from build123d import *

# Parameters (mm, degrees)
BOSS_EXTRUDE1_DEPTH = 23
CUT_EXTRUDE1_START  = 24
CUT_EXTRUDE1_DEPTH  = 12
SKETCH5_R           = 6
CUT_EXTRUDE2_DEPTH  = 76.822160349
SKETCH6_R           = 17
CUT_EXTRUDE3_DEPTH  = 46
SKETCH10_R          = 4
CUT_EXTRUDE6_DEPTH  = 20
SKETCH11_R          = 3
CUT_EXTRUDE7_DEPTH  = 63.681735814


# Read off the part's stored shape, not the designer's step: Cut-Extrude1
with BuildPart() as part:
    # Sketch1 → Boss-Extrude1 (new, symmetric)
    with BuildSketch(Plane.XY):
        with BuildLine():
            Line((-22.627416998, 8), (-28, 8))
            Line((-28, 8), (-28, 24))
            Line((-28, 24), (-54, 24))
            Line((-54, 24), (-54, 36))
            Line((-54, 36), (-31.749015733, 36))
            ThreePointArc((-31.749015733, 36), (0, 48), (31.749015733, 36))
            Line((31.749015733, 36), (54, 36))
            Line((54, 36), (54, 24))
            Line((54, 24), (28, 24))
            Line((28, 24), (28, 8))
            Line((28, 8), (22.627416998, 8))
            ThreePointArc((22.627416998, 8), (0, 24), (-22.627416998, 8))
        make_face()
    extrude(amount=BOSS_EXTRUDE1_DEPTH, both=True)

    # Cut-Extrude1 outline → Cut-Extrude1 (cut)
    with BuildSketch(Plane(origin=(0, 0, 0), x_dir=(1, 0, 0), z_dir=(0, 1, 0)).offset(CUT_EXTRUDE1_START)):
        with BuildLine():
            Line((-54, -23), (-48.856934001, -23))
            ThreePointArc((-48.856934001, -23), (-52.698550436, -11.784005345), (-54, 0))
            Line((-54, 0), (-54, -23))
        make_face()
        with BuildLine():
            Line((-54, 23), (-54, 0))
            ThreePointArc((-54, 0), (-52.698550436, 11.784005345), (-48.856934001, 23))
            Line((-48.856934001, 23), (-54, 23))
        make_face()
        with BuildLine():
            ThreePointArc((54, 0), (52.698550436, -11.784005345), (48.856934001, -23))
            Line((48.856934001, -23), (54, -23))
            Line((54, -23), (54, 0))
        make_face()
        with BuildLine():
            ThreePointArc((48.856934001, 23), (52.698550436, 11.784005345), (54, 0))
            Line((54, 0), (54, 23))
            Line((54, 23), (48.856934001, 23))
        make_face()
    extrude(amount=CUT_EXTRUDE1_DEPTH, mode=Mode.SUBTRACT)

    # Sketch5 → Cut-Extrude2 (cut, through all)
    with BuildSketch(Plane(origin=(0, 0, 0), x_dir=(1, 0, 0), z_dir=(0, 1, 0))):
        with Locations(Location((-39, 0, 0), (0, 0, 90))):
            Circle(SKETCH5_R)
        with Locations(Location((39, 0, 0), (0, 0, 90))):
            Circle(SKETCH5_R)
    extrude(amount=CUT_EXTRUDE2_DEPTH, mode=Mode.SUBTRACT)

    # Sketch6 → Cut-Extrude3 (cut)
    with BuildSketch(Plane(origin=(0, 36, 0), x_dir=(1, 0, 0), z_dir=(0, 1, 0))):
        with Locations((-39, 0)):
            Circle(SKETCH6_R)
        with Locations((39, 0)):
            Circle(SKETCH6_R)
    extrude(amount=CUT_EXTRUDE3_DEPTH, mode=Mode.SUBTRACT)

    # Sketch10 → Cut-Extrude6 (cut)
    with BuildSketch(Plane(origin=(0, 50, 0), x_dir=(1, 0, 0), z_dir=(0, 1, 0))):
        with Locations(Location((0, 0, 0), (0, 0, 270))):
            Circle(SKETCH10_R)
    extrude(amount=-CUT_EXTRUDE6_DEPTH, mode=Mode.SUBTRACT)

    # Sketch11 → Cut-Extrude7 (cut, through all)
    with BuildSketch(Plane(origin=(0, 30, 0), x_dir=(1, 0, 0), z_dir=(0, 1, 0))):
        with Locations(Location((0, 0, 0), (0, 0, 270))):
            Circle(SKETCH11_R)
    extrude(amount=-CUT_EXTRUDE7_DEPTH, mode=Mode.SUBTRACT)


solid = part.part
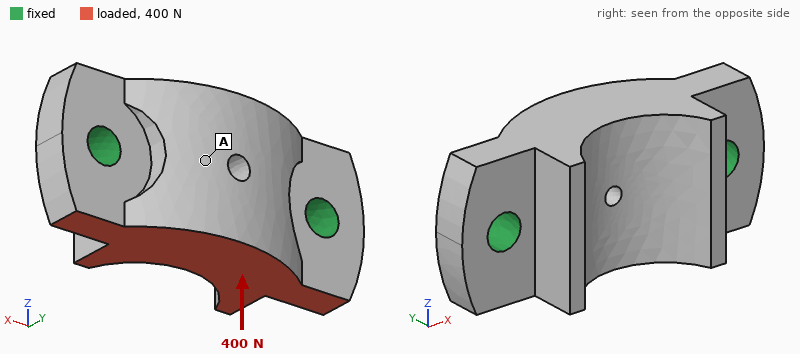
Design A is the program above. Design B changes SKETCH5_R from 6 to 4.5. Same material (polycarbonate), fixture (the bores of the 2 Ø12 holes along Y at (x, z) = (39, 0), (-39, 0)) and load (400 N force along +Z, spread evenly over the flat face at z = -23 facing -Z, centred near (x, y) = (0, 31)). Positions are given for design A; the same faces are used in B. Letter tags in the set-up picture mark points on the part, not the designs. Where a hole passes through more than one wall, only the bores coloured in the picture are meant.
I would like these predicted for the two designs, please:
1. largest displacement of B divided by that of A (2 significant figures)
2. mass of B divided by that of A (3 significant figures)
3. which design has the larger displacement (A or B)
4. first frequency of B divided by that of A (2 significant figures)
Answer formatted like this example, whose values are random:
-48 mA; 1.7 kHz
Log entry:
1.1; 1.01; B; 0.87
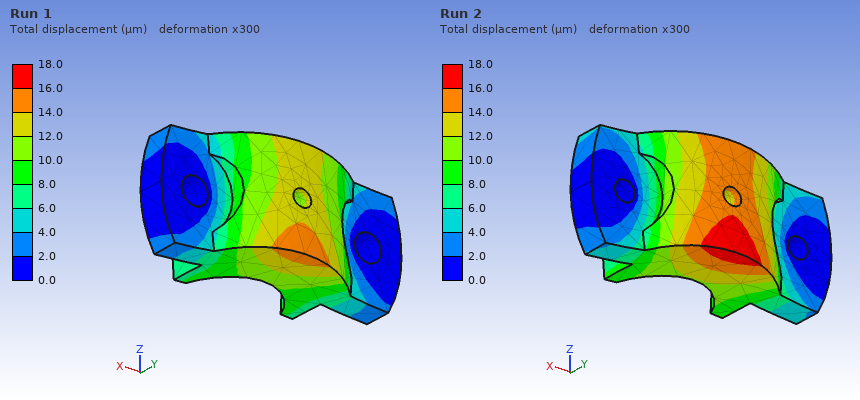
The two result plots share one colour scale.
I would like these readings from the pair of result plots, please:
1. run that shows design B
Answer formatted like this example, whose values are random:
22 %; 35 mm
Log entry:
Run 2
